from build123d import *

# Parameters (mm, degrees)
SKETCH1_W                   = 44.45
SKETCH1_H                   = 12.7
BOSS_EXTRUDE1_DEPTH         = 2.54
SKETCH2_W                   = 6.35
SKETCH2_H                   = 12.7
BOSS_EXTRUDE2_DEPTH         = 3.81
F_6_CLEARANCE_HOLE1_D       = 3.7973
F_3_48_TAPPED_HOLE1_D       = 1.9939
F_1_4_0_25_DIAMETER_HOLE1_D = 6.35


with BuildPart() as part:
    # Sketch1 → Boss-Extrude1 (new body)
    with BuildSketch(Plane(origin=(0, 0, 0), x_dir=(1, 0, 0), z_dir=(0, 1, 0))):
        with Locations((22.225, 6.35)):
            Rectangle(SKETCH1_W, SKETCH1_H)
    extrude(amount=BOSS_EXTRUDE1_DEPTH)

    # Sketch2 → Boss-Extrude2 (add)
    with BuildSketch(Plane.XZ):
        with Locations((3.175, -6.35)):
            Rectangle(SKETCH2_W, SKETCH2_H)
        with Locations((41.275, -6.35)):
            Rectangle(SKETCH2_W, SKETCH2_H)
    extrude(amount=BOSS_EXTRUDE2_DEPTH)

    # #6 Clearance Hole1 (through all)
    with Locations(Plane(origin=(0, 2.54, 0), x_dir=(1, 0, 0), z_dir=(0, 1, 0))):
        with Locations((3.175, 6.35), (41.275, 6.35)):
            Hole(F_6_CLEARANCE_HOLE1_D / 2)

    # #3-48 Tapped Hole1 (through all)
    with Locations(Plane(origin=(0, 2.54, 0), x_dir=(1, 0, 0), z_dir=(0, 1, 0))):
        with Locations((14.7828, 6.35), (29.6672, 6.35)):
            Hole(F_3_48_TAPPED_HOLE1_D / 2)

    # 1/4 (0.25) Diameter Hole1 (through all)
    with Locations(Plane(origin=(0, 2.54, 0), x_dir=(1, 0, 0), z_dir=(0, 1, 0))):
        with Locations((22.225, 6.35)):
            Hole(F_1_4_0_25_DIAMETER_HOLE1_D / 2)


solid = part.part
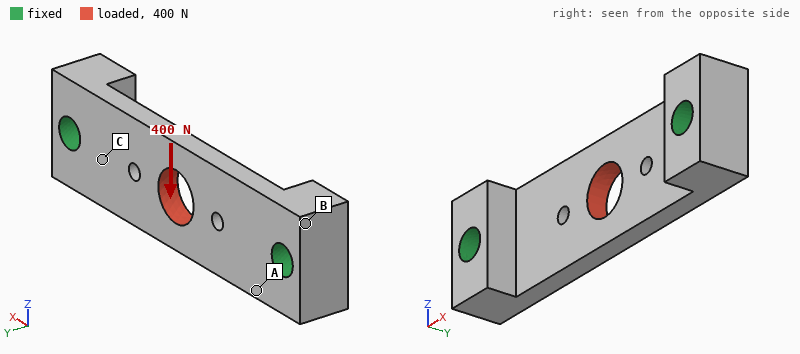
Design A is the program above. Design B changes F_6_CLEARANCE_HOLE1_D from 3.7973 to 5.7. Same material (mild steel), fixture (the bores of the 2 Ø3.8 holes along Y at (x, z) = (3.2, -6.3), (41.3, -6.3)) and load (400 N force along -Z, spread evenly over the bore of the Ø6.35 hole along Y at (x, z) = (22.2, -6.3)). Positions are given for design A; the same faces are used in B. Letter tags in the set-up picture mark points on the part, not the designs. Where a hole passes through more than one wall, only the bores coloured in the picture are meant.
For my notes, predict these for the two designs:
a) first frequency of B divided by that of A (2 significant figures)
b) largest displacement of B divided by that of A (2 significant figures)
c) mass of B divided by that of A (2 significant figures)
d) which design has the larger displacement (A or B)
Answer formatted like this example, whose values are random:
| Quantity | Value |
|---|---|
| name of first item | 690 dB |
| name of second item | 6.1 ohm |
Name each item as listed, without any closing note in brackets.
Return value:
| Quantity | Value |
|---|---|
| first frequency of B divided by that of A | 1.1 |
| largest displacement of B divided by that of A | 0.86 |
| mass of B divided by that of A | 0.90 |
| which design has the larger displacement | A |
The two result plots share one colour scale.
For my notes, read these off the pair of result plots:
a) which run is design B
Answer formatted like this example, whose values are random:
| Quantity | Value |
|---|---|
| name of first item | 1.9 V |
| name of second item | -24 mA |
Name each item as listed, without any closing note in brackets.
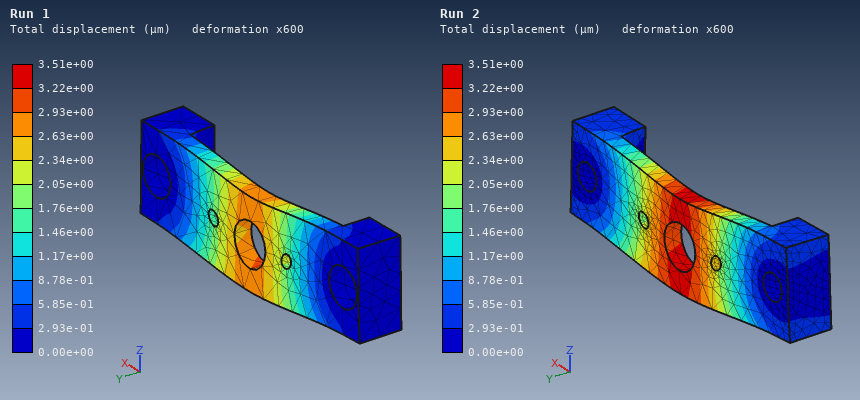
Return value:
| Quantity | Value |
|---|---|
| which run is design B | Run 1 |
